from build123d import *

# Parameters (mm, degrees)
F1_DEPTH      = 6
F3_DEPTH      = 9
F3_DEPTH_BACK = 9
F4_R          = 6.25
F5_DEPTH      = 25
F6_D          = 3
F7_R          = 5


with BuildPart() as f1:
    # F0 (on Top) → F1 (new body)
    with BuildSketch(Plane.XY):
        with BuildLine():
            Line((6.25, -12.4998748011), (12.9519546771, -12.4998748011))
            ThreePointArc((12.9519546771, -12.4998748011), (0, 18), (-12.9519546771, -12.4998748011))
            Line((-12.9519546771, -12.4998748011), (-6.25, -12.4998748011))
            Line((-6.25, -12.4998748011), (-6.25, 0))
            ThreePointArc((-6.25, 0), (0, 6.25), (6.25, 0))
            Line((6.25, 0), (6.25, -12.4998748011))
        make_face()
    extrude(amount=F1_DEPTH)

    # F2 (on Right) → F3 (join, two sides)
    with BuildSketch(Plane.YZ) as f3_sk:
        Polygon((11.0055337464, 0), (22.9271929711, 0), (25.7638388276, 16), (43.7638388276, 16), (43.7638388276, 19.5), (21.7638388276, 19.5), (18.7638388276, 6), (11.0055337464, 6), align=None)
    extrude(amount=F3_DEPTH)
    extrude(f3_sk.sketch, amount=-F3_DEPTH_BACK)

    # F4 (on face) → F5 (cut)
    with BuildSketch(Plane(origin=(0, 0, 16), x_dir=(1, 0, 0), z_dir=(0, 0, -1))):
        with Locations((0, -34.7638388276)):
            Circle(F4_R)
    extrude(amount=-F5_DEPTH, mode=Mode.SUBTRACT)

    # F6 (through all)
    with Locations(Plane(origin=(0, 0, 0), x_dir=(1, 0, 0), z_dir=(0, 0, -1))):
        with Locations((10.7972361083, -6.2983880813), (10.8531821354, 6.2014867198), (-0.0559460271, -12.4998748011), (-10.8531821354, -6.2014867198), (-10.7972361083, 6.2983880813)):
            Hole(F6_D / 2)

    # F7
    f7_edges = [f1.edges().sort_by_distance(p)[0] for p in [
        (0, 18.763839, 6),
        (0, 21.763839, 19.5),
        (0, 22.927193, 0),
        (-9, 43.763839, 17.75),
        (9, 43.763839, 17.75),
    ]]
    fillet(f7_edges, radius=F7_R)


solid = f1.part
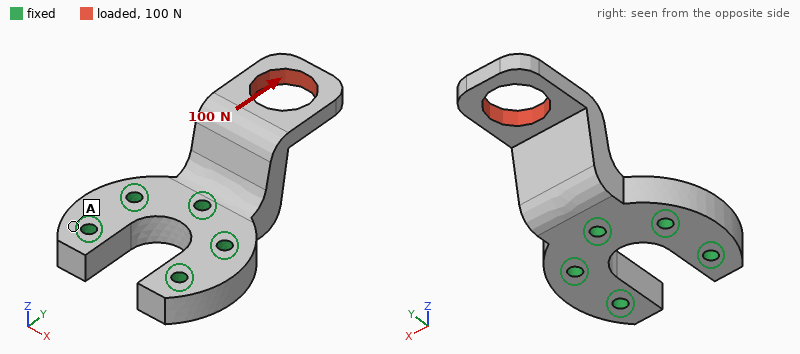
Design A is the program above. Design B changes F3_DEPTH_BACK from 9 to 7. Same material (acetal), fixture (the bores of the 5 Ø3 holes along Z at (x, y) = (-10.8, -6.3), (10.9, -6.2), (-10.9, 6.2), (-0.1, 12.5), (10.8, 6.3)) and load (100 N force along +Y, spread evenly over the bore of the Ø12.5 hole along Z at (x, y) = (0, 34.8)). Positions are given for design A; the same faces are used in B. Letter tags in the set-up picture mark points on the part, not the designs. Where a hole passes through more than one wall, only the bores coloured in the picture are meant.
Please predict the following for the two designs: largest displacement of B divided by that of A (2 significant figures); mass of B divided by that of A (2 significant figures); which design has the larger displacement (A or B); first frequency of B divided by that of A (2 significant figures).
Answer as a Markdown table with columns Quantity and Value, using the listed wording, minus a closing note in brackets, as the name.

| Quantity | Value |
|---|---|
| largest displacement of B divided by that of A | 1.1 |
| mass of B divided by that of A | 0.95 |
| which design has the larger displacement | B |
| first frequency of B divided by that of A | 1.0 |
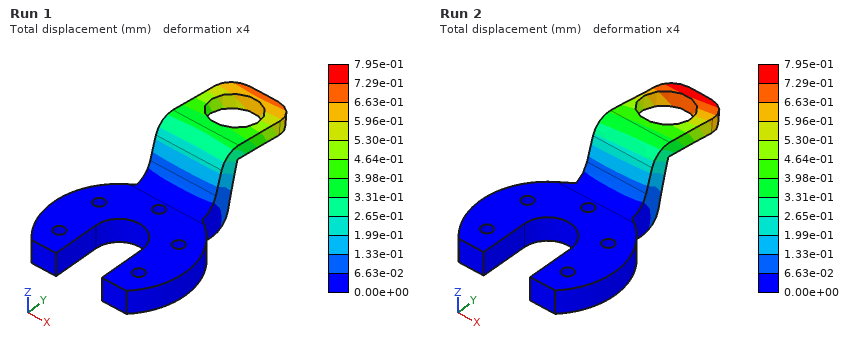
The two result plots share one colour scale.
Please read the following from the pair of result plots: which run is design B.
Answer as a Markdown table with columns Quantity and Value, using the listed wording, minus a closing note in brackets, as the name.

| Quantity | Value |
|---|---|
| which run is design B | Run 2 |
